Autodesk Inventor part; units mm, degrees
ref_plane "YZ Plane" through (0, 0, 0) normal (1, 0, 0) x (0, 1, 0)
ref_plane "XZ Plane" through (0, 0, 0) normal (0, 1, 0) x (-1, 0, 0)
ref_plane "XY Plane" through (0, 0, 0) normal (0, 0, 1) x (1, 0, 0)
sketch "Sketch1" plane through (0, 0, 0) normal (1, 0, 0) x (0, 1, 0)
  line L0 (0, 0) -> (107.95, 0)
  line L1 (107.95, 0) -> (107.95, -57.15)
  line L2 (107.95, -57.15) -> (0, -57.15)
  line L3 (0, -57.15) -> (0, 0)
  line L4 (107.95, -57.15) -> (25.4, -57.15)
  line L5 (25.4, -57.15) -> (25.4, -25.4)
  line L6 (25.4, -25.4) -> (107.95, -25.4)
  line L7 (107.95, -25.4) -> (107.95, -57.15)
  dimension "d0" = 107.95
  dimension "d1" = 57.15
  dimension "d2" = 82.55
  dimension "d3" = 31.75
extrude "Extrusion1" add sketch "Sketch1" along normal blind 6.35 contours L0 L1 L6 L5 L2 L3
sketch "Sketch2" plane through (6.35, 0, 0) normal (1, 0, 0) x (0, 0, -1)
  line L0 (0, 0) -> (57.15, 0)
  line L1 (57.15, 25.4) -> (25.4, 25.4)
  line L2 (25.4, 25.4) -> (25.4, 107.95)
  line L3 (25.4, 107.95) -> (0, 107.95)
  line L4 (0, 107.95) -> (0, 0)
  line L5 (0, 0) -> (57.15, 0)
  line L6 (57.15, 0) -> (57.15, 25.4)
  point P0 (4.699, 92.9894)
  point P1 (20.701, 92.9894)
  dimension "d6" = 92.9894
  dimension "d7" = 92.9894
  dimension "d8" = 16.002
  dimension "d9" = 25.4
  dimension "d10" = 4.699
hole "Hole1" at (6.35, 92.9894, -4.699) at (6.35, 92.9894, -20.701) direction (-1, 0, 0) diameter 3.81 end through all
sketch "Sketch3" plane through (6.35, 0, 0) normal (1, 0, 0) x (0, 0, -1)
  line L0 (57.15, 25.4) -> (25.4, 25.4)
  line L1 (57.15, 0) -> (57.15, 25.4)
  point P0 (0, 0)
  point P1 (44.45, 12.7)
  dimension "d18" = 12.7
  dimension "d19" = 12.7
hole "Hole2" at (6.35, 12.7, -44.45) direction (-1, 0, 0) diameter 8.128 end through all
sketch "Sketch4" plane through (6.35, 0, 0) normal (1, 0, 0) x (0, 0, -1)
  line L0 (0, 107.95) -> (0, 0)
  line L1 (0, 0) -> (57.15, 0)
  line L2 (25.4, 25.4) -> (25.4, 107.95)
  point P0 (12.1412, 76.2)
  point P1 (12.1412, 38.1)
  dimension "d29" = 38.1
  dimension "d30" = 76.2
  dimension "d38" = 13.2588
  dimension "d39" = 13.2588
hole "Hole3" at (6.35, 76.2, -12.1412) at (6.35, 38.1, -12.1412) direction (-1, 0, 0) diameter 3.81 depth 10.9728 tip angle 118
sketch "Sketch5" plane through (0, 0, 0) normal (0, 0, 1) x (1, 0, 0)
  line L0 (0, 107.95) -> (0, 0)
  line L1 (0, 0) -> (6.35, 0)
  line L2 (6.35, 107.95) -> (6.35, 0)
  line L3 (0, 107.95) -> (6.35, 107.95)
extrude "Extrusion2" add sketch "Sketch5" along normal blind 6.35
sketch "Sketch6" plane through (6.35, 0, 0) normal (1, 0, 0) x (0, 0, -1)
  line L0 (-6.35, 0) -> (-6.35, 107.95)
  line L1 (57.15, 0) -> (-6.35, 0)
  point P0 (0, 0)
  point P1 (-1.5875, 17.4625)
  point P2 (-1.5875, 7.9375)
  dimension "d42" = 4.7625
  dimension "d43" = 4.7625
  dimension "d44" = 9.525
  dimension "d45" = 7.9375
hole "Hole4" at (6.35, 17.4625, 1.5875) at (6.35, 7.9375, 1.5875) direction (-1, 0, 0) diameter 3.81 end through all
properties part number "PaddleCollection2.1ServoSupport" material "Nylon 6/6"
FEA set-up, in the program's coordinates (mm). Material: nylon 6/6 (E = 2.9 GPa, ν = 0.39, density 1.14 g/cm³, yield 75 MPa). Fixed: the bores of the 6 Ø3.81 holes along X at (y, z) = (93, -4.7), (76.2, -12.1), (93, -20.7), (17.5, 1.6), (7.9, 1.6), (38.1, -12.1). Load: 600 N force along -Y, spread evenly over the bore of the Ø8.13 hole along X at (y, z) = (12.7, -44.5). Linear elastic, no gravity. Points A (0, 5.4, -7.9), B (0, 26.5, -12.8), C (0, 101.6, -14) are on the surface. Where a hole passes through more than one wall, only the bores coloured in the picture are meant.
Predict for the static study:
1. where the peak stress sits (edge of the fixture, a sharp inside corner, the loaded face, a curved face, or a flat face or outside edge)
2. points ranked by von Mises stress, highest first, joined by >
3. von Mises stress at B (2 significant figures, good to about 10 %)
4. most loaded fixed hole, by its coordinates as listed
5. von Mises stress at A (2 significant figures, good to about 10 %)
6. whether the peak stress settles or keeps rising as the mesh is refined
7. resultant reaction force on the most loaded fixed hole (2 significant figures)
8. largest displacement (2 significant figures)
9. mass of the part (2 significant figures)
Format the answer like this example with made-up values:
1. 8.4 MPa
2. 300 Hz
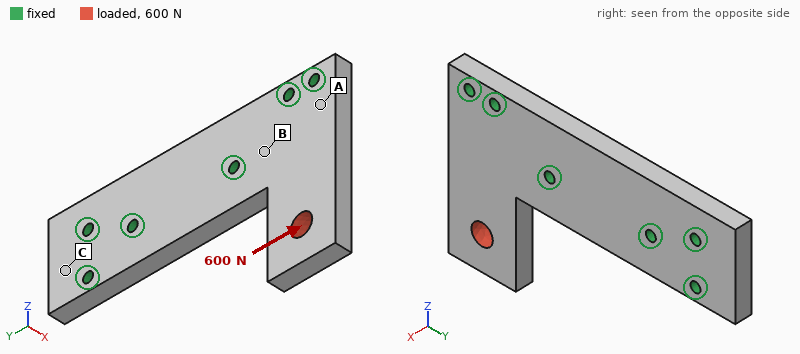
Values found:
1. a sharp inside corner
2. A > B > C
3. 5.4 MPa
4. (38.1, -12.1)
5. 9.4 MPa
6. keeps rising
7. 740 N
8. 0.59 mm
9. 30 g
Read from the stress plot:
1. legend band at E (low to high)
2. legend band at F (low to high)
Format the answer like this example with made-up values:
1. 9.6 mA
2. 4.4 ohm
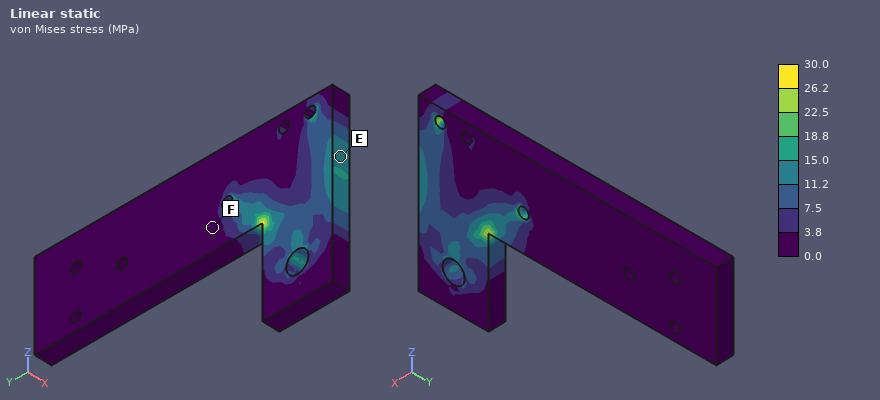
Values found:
1. 11.2 to 15.0 MPa
2. 0.0 to 3.8 MPa
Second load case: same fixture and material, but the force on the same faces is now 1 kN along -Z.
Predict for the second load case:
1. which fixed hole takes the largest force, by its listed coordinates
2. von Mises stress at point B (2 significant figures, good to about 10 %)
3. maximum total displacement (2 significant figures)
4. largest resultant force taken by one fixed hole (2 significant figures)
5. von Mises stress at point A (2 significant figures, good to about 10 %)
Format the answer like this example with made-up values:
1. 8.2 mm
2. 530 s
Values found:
1. (7.9, 1.6)
2. 2.3 MPa
3. 0.15 mm
4. 550 N
5. 7.2 MPa
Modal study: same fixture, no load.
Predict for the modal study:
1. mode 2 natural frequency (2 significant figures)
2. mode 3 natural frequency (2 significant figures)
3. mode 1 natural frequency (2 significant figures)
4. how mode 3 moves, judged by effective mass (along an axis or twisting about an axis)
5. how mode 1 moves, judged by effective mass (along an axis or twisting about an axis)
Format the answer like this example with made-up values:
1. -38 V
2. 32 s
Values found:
1. 2400 Hz
2. 2700 Hz
3. 660 Hz
4. along Y
5. along X
